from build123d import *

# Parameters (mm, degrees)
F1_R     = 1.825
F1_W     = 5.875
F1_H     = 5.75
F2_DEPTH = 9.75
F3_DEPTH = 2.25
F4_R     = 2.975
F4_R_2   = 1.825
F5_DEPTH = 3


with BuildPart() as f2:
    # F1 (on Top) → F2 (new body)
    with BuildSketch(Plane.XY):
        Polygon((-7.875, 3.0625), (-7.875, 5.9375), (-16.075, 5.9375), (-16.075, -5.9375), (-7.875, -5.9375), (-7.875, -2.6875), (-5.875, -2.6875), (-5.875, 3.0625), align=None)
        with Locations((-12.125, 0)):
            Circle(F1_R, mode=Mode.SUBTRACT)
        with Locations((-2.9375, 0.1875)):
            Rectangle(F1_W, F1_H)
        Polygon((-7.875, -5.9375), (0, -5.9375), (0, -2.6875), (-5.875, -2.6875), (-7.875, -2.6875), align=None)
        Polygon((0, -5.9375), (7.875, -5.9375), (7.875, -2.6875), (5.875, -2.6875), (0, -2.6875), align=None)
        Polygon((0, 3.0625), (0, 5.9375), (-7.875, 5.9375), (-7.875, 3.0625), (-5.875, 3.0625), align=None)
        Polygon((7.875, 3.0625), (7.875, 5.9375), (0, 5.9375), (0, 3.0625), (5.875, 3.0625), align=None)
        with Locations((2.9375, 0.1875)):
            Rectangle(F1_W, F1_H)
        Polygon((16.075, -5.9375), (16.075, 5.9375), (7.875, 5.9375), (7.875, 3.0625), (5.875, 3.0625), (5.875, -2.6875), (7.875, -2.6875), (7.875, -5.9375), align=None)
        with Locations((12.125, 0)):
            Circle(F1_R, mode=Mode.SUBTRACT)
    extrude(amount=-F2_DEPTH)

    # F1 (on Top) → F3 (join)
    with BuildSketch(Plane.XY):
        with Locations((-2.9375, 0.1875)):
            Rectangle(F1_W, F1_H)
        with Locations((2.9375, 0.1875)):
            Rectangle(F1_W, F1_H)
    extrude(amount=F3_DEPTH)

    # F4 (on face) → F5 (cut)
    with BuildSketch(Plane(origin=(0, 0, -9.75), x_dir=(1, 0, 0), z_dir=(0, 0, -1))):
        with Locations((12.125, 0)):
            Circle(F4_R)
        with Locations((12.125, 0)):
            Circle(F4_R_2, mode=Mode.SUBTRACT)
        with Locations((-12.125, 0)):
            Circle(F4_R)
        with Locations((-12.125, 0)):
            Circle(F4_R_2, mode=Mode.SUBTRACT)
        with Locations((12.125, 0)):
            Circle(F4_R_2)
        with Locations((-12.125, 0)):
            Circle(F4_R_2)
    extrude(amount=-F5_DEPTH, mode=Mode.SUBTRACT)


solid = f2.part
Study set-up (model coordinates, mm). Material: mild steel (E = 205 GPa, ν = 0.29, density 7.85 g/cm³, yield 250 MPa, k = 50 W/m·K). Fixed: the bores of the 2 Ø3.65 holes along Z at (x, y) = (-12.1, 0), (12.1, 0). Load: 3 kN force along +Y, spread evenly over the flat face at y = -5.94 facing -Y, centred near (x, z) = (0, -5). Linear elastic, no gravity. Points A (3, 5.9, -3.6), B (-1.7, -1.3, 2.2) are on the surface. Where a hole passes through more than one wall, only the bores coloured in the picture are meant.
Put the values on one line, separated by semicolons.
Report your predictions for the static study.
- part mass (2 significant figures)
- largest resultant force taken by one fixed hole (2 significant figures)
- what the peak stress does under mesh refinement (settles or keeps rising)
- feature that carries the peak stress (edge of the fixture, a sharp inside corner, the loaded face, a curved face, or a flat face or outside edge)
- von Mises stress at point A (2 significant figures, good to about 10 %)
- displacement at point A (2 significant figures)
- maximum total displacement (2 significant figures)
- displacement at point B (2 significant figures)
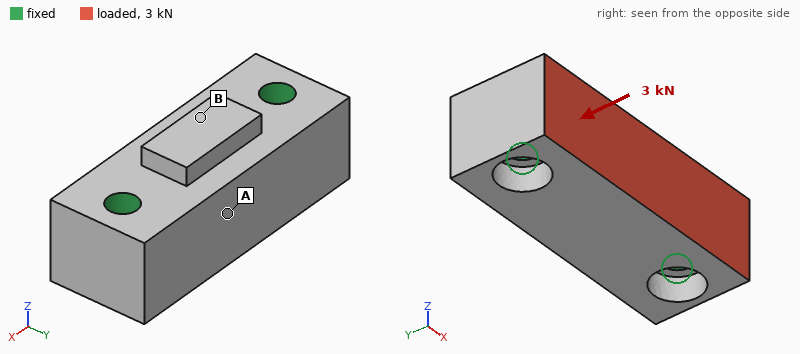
28 g; 1.5 kN; keeps rising; edge of the fixture; 17 MPa; 1.4 µm; 2.4 µm; 1.0 µm
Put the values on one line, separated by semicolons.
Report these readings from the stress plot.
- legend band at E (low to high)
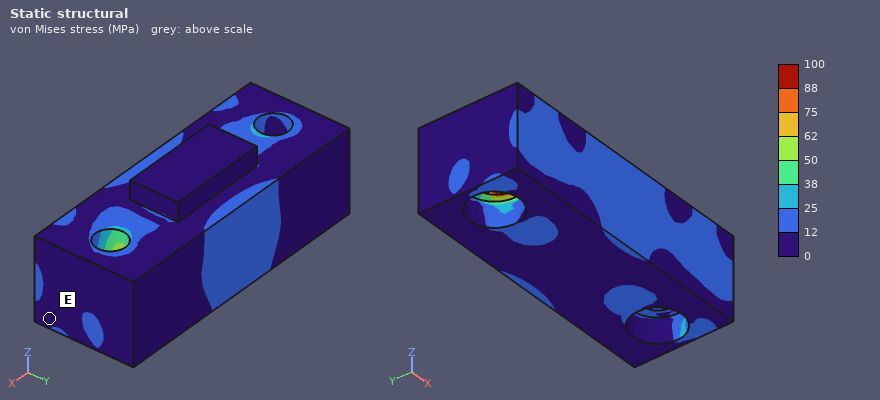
0 to 12 MPa
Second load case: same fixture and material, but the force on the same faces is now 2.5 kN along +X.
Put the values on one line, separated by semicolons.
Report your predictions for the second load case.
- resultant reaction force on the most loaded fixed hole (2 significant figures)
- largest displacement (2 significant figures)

1.4 kN; 1.6 µm
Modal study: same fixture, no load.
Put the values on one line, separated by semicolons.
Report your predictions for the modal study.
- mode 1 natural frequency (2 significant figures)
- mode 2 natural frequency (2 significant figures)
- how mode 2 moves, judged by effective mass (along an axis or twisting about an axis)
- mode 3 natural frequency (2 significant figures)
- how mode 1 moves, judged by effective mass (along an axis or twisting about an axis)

40 kHz; 43 kHz; along Z; 45 kHz; along Y
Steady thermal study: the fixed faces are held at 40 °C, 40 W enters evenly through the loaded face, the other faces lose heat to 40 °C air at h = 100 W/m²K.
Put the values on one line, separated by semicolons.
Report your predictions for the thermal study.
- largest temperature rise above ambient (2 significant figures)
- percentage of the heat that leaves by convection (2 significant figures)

30 K; 4.0 %
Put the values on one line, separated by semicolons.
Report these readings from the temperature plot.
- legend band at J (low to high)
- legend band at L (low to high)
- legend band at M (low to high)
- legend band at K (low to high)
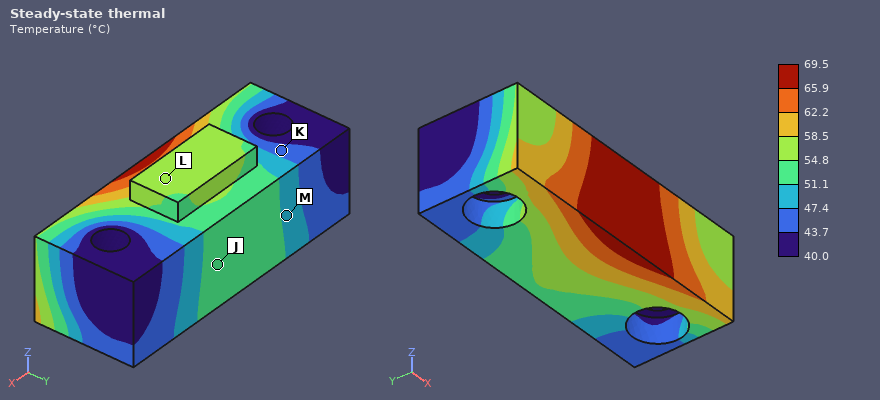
51.1 to 54.8 °C; 54.8 to 58.5 °C; 47.4 to 51.1 °C; 43.7 to 47.4 °C
